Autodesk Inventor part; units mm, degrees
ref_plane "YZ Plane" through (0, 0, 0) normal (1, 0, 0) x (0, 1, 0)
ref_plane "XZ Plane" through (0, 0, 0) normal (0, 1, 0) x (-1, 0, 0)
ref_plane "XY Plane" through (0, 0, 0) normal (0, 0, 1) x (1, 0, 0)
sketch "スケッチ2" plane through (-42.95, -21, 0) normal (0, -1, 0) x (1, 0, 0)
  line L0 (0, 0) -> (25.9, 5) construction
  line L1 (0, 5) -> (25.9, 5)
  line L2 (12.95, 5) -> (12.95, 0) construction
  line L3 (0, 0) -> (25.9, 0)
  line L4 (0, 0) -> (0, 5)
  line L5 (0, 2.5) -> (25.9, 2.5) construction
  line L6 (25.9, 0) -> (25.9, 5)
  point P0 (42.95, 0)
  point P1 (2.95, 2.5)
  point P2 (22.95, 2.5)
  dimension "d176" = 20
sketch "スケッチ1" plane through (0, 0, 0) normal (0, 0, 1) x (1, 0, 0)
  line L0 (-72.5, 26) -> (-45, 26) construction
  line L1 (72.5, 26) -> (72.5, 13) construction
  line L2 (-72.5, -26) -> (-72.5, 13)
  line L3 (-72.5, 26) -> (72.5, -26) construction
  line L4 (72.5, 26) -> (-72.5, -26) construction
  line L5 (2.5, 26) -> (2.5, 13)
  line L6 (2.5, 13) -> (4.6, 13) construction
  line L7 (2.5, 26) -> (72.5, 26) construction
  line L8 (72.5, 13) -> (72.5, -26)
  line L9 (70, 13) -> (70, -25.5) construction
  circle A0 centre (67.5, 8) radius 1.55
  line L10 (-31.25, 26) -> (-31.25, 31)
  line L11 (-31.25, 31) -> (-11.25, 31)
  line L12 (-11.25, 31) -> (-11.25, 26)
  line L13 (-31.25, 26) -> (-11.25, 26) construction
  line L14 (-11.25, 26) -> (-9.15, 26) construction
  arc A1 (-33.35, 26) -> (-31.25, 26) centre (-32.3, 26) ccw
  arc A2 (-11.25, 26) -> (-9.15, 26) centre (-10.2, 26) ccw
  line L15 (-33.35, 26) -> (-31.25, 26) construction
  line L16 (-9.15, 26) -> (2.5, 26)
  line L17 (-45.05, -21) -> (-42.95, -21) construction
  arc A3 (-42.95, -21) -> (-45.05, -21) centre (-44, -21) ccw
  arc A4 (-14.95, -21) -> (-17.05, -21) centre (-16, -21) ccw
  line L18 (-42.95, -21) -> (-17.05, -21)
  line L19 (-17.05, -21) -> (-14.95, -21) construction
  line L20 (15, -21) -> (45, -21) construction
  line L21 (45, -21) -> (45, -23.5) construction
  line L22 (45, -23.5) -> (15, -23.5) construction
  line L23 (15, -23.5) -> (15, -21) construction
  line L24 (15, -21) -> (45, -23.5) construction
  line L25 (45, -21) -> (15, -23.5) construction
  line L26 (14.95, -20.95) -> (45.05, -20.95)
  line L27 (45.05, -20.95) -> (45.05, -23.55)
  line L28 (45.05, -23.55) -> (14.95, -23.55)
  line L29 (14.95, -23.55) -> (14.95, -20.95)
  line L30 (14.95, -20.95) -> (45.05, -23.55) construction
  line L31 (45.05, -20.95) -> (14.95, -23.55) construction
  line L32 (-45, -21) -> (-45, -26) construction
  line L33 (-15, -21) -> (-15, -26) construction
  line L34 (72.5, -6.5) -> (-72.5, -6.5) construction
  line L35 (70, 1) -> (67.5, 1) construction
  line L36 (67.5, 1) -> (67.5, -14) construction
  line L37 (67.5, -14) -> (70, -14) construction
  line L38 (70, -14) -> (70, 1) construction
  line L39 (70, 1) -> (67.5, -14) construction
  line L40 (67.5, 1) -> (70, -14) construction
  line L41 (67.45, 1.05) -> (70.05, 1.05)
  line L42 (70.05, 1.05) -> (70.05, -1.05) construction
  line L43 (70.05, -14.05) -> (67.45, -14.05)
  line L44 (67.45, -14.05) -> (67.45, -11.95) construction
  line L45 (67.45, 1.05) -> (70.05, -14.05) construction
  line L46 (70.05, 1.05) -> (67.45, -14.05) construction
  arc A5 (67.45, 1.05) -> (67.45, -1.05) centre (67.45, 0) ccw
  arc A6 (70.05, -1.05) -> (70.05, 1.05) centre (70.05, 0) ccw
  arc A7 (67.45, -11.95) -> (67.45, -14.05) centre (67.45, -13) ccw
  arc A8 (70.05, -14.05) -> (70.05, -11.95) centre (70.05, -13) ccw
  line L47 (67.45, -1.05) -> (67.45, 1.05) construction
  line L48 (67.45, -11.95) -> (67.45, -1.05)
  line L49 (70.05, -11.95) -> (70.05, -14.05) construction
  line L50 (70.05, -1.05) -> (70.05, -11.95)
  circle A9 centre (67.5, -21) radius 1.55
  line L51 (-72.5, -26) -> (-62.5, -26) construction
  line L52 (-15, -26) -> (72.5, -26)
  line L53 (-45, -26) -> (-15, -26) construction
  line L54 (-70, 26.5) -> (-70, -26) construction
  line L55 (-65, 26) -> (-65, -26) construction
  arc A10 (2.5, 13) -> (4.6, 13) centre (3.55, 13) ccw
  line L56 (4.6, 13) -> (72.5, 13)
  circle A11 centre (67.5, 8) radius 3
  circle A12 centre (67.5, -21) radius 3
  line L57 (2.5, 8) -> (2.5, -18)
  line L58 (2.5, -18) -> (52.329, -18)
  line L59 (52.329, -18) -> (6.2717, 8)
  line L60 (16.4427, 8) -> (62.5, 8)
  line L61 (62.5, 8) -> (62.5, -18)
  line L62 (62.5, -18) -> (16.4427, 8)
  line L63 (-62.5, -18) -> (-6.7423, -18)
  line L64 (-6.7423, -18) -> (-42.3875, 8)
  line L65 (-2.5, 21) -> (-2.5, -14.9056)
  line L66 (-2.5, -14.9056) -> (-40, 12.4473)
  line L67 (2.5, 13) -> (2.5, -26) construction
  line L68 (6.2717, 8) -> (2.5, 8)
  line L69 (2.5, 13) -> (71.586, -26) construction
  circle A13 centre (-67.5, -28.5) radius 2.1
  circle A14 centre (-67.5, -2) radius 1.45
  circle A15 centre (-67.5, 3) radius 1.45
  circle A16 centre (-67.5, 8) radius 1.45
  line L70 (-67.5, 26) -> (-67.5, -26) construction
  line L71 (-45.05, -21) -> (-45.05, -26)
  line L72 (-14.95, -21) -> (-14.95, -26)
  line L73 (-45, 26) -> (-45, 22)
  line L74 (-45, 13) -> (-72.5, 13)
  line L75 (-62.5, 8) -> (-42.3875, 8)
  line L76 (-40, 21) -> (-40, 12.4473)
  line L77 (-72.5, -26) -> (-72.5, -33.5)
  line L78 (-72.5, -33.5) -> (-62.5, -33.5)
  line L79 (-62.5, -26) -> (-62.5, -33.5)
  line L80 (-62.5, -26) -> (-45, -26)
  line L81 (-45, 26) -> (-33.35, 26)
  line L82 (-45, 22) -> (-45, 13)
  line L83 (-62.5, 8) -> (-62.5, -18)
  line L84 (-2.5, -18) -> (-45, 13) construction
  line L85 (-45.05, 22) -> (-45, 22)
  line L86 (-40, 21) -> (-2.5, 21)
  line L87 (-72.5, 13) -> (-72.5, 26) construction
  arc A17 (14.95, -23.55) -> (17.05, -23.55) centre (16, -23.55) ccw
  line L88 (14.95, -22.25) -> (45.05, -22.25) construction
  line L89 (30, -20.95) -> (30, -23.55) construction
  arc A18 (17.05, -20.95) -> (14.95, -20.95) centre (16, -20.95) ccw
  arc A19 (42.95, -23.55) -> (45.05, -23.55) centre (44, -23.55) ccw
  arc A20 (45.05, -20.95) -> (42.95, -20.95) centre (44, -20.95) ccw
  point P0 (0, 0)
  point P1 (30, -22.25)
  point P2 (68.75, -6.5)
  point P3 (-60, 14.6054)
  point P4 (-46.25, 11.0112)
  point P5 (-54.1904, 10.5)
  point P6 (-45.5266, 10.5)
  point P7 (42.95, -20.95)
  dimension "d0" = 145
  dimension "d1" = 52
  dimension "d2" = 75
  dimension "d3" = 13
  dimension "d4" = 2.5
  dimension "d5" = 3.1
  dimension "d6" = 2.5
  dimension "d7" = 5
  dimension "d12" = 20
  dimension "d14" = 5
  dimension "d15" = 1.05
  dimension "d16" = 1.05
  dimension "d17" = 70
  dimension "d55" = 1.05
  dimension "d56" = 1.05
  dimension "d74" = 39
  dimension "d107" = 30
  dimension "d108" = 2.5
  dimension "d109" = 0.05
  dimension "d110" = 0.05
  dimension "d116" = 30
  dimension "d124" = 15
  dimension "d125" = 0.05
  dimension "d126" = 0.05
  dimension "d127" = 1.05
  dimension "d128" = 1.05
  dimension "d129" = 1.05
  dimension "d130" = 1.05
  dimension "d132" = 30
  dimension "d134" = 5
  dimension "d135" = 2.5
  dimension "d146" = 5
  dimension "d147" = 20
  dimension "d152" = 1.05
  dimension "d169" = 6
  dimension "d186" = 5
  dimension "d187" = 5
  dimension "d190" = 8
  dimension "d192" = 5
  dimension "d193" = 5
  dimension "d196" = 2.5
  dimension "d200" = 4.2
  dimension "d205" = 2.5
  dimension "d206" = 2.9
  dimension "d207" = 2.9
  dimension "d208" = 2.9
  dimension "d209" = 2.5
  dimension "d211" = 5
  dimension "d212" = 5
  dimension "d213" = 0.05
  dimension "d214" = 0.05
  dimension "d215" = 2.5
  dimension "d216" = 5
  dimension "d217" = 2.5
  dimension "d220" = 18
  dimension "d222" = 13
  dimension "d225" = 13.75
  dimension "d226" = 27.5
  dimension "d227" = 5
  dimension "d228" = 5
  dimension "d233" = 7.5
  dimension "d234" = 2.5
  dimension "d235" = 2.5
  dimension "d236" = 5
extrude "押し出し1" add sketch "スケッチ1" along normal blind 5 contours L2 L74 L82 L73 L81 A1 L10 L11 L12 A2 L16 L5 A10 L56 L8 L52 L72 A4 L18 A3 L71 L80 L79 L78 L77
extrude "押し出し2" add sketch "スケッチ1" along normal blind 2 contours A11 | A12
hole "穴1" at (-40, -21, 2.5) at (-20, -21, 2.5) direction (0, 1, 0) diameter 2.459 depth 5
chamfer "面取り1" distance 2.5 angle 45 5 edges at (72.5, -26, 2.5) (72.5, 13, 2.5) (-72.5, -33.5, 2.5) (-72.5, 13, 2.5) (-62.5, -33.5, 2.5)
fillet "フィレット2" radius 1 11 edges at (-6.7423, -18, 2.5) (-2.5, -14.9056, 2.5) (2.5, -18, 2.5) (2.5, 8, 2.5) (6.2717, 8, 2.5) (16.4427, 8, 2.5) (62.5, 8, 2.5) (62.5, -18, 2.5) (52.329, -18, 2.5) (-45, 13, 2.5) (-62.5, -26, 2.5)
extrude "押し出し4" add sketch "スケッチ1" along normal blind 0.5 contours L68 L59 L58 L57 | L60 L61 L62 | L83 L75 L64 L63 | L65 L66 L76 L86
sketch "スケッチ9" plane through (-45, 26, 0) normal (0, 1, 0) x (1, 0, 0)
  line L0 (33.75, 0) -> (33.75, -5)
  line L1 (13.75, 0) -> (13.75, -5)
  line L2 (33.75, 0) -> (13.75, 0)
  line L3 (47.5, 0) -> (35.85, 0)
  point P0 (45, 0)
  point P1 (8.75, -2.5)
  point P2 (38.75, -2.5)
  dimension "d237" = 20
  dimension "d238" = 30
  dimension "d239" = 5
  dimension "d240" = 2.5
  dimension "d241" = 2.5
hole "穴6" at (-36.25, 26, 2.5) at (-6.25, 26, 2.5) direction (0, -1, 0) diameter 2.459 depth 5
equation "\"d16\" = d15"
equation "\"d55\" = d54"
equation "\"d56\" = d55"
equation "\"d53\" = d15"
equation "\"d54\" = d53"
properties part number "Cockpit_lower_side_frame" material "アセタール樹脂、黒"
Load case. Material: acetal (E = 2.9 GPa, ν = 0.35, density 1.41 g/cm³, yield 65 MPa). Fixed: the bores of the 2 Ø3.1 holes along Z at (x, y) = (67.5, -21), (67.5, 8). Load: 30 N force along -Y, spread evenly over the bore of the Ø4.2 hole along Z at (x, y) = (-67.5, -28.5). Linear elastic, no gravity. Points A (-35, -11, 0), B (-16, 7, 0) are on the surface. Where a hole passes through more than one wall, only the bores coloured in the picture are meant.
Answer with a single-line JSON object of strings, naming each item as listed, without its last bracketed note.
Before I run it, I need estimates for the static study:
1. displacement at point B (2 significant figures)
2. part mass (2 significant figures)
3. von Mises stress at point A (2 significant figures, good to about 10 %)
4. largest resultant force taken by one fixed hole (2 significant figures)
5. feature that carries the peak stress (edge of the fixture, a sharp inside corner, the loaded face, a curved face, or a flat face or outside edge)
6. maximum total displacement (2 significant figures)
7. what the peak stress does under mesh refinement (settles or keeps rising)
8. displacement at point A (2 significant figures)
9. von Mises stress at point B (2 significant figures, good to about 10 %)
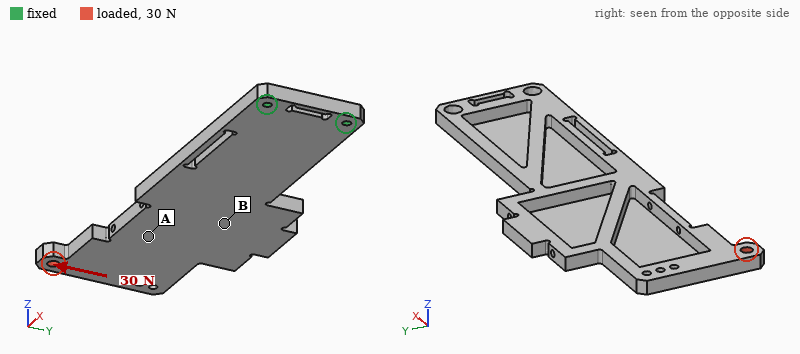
{"displacement at point B": "0.42 mm", "part mass": "23 g", "von Mises stress at point A": "1.6 MPa", "largest resultant force taken by one fixed hole": "130 N", "feature that carries the peak stress": "edge of the fixture", "maximum total displacement": "1.7 mm", "what the peak stress does under mesh refinement": "keeps rising", "displacement at point A": "0.72 mm", "von Mises stress at point B": "4.7 MPa"}
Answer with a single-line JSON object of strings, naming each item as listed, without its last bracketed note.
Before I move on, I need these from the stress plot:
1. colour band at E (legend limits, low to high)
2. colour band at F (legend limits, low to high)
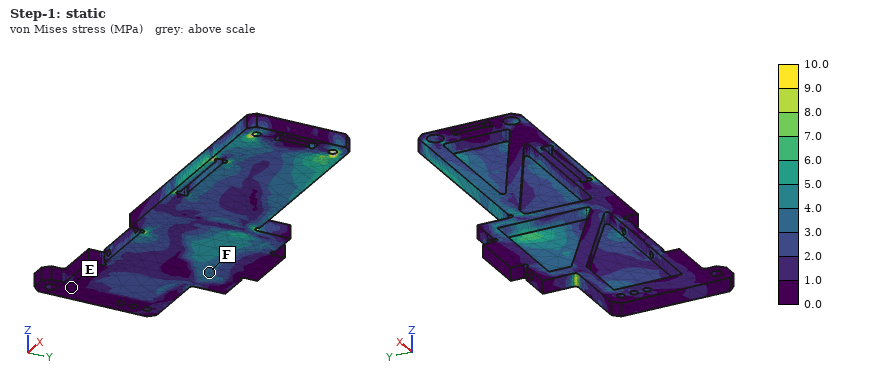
{"colour band at E": "0.0 to 1.0 MPa", "colour band at F": "3.0 to 4.0 MPa"}
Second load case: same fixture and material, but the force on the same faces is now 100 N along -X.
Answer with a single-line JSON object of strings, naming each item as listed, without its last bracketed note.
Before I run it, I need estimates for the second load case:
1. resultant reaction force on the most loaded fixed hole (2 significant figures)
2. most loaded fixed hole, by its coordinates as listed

{"resultant reaction force on the most loaded fixed hole": "120 N", "most loaded fixed hole, by its coordinates as listed": "(67.5, -21)"}
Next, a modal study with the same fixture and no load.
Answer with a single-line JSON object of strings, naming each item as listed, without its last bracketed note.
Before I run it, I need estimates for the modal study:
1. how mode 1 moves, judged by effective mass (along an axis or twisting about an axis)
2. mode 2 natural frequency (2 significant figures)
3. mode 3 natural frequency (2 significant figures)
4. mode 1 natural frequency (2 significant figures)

{"how mode 1 moves, judged by effective mass": "along Z", "mode 2 natural frequency": "170 Hz", "mode 3 natural frequency": "290 Hz", "mode 1 natural frequency": "45 Hz"}
